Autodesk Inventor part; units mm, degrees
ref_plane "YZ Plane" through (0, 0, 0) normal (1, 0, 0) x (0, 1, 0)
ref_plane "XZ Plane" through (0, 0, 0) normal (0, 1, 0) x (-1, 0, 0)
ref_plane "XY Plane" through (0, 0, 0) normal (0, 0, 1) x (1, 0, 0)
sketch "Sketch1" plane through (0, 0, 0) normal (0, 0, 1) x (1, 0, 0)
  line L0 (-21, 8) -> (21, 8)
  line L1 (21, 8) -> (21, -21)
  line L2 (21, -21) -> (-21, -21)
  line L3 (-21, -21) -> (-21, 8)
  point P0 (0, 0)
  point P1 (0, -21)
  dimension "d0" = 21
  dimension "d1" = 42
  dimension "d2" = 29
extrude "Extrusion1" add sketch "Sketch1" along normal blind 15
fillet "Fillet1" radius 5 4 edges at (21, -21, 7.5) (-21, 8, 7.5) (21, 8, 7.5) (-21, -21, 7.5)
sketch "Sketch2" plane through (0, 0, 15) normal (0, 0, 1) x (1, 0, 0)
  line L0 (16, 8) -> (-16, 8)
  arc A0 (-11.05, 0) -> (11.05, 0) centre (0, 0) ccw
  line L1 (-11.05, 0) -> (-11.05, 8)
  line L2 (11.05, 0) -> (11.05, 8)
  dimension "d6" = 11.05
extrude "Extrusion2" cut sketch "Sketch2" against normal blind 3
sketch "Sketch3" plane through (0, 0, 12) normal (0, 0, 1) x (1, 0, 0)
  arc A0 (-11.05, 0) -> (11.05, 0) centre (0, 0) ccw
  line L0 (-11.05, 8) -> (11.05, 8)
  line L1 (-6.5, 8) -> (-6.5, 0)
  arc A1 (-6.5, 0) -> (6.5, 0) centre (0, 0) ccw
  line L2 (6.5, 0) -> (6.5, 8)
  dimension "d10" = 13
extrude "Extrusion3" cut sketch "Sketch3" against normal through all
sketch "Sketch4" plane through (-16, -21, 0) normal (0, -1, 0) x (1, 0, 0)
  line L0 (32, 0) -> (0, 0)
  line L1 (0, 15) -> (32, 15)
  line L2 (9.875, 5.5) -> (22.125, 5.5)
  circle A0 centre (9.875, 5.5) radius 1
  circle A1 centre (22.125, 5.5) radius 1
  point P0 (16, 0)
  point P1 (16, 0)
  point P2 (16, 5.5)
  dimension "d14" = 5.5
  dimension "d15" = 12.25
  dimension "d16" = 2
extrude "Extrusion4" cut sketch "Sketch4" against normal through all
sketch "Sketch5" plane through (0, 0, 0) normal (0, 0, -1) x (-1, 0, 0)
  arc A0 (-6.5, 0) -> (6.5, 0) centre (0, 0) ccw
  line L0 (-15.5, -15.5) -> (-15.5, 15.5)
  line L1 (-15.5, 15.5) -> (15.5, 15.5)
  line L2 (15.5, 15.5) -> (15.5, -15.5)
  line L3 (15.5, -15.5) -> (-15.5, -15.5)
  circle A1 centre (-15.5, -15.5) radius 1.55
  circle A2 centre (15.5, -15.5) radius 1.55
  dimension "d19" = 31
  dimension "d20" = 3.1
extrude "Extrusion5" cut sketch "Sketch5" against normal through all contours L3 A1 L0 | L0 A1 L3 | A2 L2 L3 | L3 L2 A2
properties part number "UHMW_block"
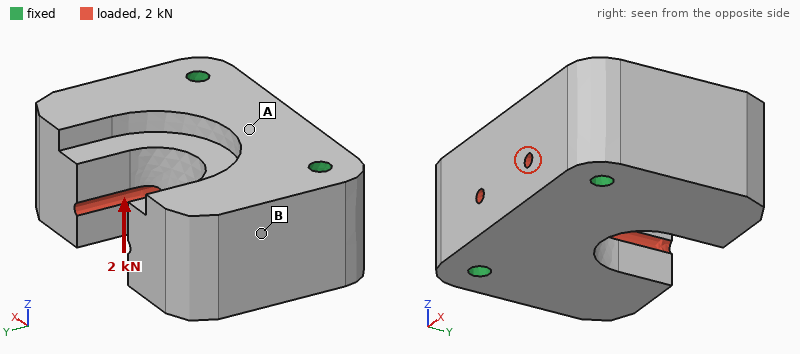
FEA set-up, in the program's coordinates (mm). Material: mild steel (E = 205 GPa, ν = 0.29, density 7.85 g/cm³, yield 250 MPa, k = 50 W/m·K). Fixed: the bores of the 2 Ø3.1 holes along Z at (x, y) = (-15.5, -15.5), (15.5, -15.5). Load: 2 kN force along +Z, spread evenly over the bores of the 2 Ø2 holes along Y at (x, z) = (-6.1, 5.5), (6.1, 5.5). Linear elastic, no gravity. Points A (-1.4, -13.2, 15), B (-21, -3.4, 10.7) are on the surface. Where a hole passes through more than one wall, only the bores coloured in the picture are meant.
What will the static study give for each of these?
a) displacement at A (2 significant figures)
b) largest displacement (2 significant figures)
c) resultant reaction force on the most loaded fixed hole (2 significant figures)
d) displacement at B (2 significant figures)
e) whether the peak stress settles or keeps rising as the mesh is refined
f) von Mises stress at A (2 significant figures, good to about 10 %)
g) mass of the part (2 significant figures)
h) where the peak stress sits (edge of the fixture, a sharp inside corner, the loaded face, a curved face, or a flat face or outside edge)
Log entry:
1.1 µm
2.9 µm
1.0 kN
0.66 µm
keeps rising
8.4 MPa
110 g
edge of the fixture
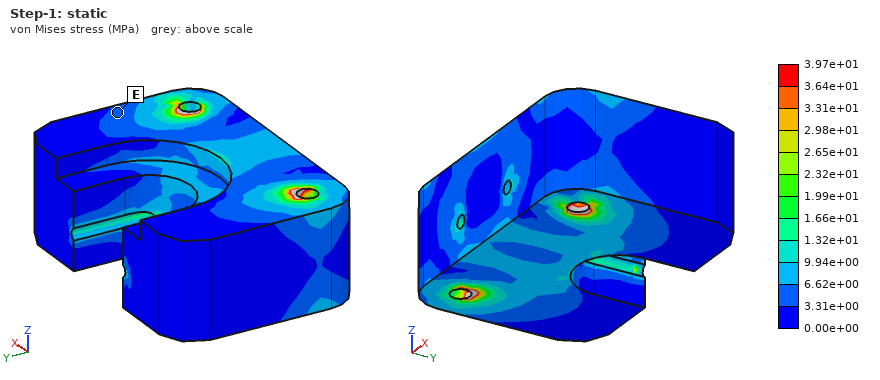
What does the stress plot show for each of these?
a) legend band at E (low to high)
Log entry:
3.31e+00 to 6.62e+00 MPa
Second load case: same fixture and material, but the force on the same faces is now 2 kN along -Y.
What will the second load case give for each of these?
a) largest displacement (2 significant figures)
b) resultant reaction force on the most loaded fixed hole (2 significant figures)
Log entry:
2.5 µm
1.1 kN
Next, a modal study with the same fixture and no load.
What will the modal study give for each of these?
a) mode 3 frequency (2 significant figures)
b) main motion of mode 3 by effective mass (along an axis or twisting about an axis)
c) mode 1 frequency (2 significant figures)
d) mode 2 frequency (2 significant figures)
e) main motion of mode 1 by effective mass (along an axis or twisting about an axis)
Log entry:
19 kHz
twisting about Y
16 kHz
17 kHz
along Z
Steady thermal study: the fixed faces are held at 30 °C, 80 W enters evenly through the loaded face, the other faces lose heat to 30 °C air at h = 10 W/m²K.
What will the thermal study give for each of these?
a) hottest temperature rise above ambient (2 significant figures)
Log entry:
49 K
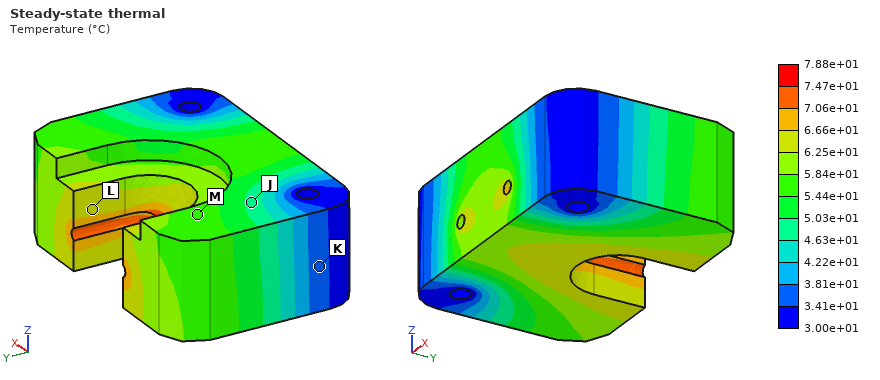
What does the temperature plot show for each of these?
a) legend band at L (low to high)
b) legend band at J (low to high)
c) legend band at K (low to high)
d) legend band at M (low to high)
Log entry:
6.25e+01 to 6.66e+01 °C
4.63e+01 to 5.03e+01 °C
3.41e+01 to 3.81e+01 °C
5.44e+01 to 5.84e+01 °C
